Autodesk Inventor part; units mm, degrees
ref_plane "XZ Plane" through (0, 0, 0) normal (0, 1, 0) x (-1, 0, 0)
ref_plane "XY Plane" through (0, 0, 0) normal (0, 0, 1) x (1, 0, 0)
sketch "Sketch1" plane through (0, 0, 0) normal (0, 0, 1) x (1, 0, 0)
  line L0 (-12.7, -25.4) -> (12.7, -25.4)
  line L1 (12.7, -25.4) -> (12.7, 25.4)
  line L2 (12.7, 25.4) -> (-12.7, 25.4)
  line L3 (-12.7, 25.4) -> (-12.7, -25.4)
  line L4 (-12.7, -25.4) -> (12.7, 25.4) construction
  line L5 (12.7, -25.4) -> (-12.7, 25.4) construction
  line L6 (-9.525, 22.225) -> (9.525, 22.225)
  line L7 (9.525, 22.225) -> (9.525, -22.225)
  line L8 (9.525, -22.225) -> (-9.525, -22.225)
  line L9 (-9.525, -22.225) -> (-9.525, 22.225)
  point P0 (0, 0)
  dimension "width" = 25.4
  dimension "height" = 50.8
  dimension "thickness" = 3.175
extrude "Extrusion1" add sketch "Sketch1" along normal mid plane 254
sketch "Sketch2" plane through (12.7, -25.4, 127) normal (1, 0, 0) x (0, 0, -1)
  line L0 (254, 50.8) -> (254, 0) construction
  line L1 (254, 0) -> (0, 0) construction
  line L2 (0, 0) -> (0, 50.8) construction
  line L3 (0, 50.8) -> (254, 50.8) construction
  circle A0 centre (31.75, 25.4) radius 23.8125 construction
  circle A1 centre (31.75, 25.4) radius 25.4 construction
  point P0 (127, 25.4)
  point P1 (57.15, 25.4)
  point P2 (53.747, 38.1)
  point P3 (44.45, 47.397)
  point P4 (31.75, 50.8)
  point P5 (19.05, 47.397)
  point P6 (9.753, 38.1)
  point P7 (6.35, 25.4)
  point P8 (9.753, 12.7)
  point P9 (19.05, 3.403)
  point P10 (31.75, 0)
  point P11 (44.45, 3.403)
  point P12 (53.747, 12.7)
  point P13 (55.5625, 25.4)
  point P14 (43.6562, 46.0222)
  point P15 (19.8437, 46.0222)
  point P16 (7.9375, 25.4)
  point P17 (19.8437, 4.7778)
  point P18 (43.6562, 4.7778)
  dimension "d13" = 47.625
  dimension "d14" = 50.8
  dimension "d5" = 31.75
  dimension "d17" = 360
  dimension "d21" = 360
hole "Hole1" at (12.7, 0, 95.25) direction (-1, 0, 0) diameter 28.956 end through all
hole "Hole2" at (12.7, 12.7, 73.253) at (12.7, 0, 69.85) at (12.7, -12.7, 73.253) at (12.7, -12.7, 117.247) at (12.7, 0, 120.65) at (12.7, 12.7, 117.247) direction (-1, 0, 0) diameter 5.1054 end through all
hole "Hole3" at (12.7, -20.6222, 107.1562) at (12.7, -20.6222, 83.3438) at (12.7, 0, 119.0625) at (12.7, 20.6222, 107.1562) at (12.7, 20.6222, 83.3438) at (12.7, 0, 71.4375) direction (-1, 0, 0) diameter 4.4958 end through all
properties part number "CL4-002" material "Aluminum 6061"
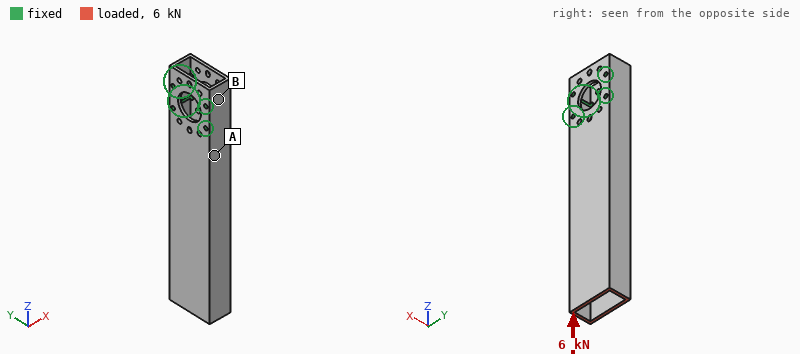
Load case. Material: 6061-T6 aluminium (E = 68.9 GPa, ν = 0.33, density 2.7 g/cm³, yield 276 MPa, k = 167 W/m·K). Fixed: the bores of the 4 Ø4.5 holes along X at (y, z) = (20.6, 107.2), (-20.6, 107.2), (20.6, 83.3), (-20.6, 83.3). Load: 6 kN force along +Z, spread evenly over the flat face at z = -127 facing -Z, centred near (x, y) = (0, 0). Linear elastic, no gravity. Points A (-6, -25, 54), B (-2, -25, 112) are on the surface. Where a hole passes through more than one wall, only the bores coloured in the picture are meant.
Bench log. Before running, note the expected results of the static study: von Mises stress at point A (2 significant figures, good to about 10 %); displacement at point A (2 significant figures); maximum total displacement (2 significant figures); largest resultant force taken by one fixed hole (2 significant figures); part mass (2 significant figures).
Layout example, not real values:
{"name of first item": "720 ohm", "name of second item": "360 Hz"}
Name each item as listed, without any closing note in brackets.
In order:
{"von Mises stress at point A": "16 MPa", "displacement at point A": "7.7 µm", "maximum total displacement": "43 µm", "largest resultant force taken by one fixed hole": "2.8 kN", "part mass": "290 g"}
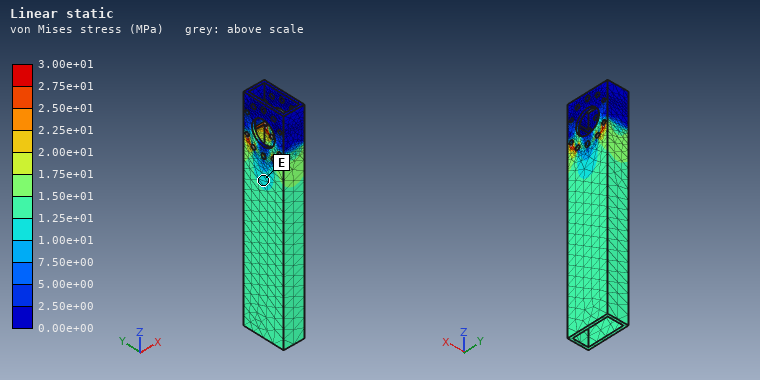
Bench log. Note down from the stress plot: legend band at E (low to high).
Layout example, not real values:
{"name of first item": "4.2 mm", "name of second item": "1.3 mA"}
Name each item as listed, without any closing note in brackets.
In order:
{"legend band at E": "1.00e+01 to 1.25e+01 MPa"}
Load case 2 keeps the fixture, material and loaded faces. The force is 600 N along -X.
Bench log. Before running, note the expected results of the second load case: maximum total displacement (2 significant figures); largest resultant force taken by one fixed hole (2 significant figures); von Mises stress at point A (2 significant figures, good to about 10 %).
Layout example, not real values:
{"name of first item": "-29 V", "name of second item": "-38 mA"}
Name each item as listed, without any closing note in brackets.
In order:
{"maximum total displacement": "0.81 mm", "largest resultant force taken by one fixed hole": "380 N", "von Mises stress at point A": "21 MPa"}
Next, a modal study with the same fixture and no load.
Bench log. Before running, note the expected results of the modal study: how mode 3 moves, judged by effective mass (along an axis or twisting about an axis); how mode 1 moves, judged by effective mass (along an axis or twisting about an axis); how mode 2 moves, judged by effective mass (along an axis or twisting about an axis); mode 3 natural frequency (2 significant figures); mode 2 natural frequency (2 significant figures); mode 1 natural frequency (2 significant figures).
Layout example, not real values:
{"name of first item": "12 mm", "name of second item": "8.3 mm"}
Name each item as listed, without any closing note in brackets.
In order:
{"how mode 3 moves, judged by effective mass": "twisting about Z", "how mode 1 moves, judged by effective mass": "along X", "how mode 2 moves, judged by effective mass": "along Y", "mode 3 natural frequency": "2500 Hz", "mode 2 natural frequency": "1000 Hz", "mode 1 natural frequency": "550 Hz"}
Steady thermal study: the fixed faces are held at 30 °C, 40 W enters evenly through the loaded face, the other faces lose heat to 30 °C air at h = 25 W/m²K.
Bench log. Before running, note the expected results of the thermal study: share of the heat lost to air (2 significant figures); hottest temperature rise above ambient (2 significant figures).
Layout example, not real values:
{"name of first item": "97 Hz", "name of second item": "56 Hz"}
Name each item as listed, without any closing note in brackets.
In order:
{"share of the heat lost to air": "76 %", "hottest temperature rise above ambient": "54 K"}
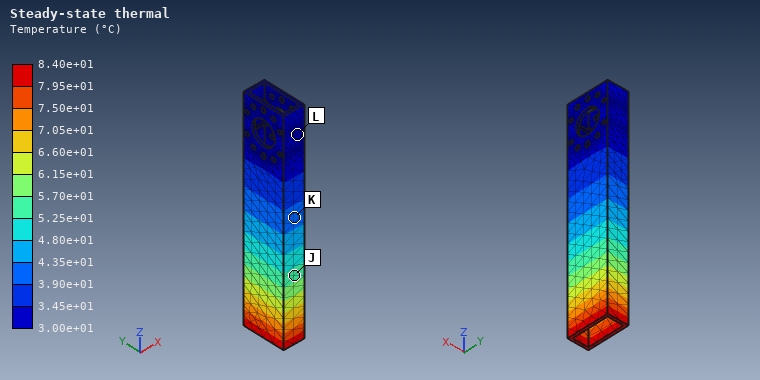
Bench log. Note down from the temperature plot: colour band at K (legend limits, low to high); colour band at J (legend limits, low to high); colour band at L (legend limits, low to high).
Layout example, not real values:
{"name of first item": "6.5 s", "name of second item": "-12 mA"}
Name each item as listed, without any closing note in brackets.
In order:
{"colour band at K": "3.90e+01 to 4.35e+01 °C", "colour band at J": "5.25e+01 to 5.70e+01 °C", "colour band at L": "3.00e+01 to 3.45e+01 °C"}
